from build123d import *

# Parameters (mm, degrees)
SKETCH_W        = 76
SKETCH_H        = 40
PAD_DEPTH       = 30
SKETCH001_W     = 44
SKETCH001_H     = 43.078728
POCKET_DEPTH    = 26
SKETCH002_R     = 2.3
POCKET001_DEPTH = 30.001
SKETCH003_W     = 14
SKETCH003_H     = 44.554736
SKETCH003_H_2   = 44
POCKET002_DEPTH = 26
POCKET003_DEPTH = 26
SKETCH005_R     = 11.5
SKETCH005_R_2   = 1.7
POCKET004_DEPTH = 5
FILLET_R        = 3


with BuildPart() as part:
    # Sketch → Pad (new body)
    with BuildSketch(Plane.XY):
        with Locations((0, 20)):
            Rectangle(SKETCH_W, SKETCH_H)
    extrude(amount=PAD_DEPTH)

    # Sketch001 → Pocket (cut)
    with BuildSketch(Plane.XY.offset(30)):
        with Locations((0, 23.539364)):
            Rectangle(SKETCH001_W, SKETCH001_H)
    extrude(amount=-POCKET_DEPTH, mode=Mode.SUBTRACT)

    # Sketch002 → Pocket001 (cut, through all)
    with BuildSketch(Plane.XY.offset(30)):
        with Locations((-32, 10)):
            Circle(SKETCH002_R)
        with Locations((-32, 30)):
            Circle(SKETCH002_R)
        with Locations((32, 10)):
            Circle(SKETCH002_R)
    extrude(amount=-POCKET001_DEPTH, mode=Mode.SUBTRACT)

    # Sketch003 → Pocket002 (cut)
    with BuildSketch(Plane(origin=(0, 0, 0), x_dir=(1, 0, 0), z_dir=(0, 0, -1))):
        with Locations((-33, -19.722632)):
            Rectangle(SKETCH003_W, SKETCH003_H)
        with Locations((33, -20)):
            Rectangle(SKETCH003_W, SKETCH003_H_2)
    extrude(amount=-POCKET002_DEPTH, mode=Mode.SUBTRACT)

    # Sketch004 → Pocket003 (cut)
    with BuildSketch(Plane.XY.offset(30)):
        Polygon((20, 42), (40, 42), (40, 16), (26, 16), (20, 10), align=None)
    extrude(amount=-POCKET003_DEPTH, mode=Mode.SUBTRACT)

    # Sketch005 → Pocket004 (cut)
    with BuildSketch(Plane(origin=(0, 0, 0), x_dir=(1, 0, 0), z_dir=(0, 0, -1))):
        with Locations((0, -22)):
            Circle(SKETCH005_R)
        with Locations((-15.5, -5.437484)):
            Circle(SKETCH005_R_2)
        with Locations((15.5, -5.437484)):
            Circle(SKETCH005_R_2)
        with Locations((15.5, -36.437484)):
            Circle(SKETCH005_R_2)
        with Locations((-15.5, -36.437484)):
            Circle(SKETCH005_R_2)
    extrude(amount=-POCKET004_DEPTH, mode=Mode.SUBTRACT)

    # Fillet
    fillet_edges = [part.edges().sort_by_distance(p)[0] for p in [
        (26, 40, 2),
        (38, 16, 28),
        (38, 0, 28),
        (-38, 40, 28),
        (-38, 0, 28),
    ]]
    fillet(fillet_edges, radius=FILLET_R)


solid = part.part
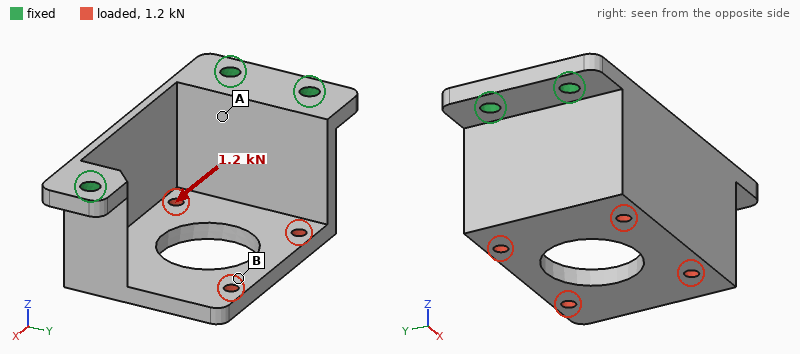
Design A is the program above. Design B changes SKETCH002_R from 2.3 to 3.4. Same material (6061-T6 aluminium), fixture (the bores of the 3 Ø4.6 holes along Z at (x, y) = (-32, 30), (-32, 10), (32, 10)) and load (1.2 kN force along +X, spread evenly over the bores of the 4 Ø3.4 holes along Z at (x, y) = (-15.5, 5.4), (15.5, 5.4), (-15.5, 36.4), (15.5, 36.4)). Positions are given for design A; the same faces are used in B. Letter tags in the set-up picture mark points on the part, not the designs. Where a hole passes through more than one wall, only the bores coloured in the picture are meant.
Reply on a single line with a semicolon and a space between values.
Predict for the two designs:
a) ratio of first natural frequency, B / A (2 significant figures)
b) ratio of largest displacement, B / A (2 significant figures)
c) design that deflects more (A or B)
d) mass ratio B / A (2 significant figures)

1.1; 0.87; A; 0.99
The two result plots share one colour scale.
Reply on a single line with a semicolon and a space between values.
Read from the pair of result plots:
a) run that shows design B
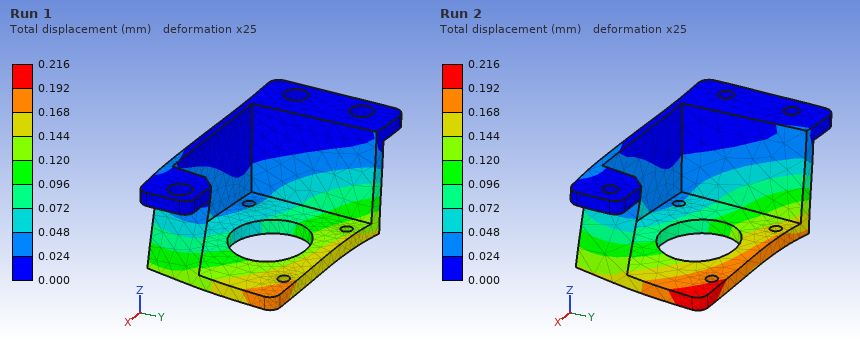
Run 1
